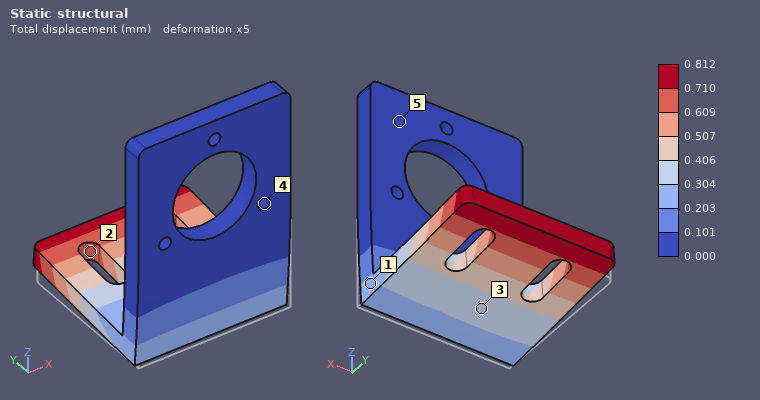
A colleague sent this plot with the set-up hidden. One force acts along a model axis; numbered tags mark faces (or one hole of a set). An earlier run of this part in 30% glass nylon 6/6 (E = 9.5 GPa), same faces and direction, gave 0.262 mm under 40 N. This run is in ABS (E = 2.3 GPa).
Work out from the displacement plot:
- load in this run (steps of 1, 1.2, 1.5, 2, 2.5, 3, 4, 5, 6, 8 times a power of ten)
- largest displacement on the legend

30 N
0.812 mm
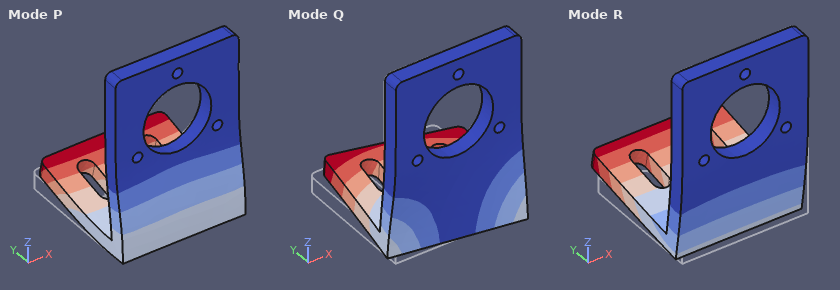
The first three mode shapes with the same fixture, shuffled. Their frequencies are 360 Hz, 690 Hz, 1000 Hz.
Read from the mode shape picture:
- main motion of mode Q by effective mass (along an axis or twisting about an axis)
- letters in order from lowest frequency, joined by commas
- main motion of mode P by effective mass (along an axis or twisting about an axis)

along X
R, Q, P
along Y
